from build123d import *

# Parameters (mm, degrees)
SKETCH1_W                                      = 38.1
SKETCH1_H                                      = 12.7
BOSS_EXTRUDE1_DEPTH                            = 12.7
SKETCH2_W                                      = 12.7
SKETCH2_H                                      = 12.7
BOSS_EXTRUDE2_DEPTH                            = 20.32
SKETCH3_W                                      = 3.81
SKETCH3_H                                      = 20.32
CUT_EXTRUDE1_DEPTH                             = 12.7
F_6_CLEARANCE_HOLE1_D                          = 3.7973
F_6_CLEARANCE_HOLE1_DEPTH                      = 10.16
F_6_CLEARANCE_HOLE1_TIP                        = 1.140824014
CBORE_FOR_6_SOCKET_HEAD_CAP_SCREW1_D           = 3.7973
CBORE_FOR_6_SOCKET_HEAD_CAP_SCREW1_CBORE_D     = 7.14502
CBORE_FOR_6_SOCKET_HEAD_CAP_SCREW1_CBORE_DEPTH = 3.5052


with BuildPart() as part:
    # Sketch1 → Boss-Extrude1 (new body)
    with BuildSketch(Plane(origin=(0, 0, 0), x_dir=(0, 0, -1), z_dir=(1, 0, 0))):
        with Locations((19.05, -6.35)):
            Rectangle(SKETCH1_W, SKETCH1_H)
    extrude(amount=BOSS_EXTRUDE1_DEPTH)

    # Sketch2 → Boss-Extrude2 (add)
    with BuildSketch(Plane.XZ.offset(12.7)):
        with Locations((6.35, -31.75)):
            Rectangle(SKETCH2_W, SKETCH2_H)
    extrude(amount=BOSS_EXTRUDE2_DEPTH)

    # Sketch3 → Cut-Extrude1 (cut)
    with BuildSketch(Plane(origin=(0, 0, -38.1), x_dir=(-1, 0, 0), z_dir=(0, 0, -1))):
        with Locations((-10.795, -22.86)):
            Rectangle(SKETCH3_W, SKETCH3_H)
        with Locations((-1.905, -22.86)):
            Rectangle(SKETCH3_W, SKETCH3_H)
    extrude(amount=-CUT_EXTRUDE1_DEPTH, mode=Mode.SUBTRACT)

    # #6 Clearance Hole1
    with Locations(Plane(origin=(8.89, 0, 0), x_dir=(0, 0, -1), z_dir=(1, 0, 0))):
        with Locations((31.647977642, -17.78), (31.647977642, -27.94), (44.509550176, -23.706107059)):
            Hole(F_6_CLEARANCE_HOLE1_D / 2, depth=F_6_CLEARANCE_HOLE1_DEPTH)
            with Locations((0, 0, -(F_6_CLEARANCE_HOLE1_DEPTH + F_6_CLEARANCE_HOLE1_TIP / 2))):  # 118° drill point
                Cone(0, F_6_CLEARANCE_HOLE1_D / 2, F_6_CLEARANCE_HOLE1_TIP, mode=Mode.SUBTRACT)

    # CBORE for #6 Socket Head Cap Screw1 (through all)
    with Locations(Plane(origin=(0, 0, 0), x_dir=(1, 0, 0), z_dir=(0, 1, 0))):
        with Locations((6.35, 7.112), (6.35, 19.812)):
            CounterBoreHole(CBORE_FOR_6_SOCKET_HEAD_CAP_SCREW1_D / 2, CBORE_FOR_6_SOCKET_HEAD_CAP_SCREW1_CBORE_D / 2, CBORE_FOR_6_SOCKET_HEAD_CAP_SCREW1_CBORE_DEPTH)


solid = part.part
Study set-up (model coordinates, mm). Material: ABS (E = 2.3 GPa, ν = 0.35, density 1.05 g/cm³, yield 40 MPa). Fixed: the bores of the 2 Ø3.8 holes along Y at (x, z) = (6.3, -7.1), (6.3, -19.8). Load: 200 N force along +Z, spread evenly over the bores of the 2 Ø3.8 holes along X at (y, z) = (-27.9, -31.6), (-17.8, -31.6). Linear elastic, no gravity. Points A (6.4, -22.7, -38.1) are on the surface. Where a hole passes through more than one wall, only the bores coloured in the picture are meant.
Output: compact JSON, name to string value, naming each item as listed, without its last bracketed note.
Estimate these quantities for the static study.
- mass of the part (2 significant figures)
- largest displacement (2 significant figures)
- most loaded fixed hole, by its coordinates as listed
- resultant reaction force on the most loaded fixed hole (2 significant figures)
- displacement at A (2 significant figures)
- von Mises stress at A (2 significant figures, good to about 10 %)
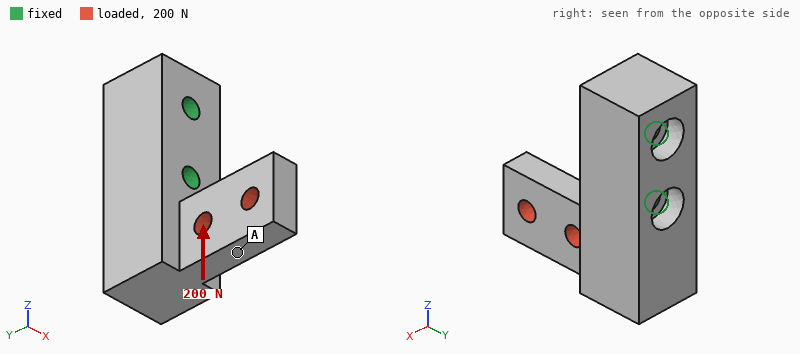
{"mass of the part": "7.2 g", "largest displacement": "0.52 mm", "most loaded fixed hole, by its coordinates as listed": "(6.3, -19.8)", "resultant reaction force on the most loaded fixed hole": "240 N", "displacement at A": "0.33 mm", "von Mises stress at A": "2.9 MPa"}
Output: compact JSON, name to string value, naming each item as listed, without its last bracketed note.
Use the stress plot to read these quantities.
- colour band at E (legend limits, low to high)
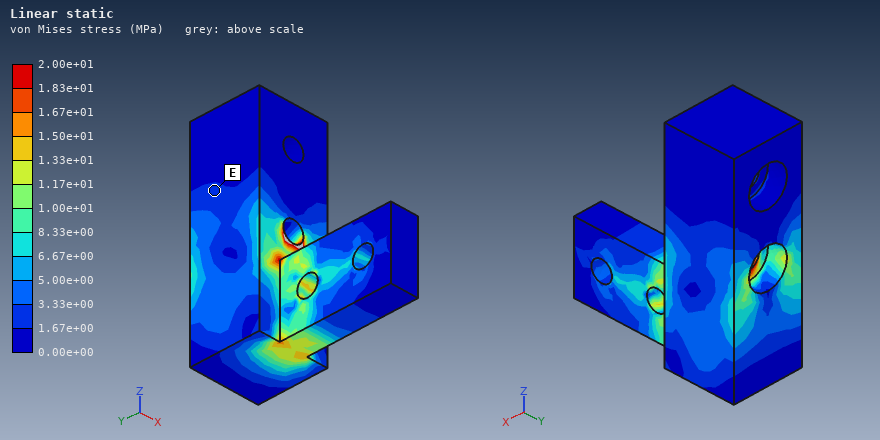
{"colour band at E": "1.67e+00 to 3.33e+00 MPa"}
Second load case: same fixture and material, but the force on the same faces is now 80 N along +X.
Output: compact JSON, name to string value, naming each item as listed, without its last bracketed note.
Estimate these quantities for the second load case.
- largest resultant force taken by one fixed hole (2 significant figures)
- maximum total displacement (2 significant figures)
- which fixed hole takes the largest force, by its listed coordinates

{"largest resultant force taken by one fixed hole": "120 N", "maximum total displacement": "0.57 mm", "which fixed hole takes the largest force, by its listed coordinates": "(6.3, -19.8)"}
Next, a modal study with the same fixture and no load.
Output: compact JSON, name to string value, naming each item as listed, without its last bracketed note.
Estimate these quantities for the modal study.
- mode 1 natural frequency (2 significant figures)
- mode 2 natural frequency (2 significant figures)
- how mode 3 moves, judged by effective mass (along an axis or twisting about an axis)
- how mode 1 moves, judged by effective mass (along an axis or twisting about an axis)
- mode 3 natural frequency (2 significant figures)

{"mode 1 natural frequency": "2100 Hz", "mode 2 natural frequency": "3000 Hz", "how mode 3 moves, judged by effective mass": "along X", "how mode 1 moves, judged by effective mass": "along X", "mode 3 natural frequency": "4800 Hz"}
